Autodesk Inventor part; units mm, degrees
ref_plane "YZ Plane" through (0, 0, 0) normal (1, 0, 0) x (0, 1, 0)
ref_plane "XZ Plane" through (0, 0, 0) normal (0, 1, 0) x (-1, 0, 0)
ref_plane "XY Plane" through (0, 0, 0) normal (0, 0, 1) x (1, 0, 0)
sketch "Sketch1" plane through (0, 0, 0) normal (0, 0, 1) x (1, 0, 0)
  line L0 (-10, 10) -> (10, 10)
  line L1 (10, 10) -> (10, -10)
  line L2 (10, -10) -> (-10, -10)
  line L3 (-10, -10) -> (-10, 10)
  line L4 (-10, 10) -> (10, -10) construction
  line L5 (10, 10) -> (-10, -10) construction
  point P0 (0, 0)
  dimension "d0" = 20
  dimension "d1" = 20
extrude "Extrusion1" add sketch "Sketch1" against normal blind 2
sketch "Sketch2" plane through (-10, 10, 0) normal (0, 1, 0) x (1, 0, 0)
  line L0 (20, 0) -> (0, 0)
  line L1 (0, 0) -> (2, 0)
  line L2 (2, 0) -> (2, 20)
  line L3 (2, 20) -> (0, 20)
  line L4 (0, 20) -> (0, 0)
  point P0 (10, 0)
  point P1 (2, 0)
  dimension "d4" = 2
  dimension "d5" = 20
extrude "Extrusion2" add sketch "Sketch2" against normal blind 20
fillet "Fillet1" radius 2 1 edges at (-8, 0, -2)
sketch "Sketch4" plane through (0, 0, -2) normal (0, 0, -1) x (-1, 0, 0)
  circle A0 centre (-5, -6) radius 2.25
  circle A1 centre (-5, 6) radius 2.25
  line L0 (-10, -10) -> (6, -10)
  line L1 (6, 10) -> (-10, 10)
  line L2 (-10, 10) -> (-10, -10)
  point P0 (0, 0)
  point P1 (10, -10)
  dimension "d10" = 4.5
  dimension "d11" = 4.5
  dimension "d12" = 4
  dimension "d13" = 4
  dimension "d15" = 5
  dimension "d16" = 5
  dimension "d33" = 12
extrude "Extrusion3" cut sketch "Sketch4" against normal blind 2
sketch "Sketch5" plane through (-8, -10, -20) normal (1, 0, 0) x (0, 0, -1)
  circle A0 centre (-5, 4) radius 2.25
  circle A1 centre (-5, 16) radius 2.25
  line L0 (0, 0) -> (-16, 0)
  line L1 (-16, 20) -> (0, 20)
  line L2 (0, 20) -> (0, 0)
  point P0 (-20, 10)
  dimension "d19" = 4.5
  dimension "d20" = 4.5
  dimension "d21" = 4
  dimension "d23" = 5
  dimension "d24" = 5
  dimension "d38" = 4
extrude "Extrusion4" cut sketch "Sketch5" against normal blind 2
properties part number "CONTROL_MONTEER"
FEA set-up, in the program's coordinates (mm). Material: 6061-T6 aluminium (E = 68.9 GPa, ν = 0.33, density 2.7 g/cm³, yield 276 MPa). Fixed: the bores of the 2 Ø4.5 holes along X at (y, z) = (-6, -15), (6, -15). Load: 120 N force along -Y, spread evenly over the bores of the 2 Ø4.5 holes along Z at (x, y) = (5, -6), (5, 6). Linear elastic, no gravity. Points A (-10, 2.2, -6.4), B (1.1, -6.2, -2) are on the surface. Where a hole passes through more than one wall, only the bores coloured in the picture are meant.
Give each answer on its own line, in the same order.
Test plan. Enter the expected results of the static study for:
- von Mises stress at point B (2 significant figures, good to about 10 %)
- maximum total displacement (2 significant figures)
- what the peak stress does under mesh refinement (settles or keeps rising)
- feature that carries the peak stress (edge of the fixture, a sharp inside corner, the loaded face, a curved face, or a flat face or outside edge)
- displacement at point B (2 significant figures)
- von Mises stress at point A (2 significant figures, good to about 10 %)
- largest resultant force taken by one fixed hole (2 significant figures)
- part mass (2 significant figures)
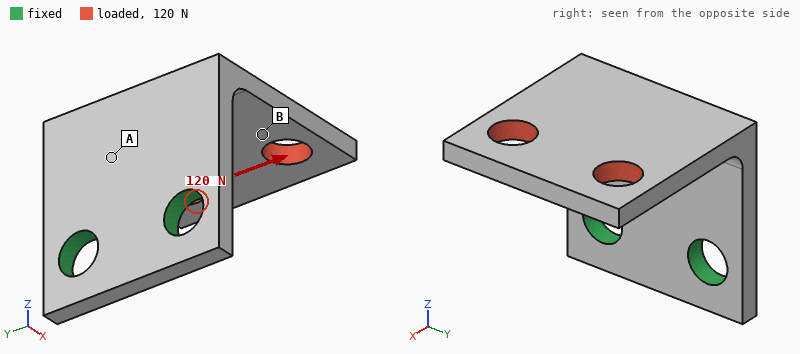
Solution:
16 MPa
0.15 mm
keeps rising
edge of the fixture
0.083 mm
53 MPa
170 N
3.8 g
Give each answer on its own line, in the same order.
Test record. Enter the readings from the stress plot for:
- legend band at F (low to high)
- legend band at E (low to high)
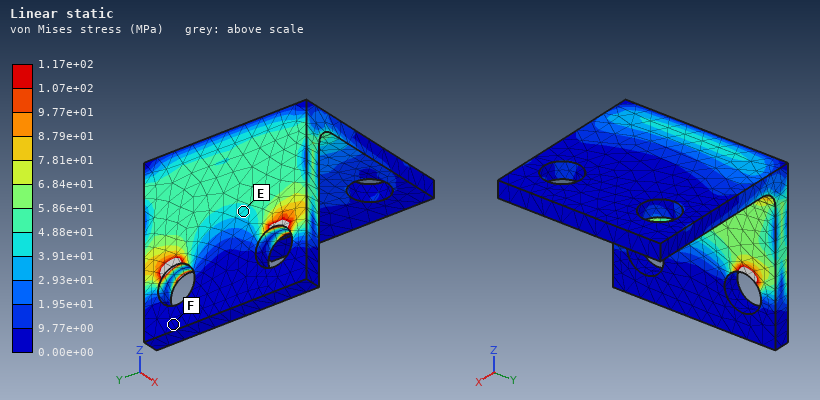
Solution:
0.00e+00 to 9.77e+00 MPa
3.91e+01 to 4.88e+01 MPa
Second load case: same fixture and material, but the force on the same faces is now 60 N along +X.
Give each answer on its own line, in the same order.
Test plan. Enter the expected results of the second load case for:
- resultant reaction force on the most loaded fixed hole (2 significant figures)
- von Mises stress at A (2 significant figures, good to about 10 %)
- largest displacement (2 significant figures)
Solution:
30 N
21 MPa
0.10 mm
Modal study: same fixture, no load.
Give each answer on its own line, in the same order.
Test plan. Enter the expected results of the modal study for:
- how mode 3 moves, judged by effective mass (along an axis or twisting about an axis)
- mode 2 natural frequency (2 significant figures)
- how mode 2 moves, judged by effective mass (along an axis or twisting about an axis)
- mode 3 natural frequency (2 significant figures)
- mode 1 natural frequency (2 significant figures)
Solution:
along X
4600 Hz
along Y
7300 Hz
2400 Hz
